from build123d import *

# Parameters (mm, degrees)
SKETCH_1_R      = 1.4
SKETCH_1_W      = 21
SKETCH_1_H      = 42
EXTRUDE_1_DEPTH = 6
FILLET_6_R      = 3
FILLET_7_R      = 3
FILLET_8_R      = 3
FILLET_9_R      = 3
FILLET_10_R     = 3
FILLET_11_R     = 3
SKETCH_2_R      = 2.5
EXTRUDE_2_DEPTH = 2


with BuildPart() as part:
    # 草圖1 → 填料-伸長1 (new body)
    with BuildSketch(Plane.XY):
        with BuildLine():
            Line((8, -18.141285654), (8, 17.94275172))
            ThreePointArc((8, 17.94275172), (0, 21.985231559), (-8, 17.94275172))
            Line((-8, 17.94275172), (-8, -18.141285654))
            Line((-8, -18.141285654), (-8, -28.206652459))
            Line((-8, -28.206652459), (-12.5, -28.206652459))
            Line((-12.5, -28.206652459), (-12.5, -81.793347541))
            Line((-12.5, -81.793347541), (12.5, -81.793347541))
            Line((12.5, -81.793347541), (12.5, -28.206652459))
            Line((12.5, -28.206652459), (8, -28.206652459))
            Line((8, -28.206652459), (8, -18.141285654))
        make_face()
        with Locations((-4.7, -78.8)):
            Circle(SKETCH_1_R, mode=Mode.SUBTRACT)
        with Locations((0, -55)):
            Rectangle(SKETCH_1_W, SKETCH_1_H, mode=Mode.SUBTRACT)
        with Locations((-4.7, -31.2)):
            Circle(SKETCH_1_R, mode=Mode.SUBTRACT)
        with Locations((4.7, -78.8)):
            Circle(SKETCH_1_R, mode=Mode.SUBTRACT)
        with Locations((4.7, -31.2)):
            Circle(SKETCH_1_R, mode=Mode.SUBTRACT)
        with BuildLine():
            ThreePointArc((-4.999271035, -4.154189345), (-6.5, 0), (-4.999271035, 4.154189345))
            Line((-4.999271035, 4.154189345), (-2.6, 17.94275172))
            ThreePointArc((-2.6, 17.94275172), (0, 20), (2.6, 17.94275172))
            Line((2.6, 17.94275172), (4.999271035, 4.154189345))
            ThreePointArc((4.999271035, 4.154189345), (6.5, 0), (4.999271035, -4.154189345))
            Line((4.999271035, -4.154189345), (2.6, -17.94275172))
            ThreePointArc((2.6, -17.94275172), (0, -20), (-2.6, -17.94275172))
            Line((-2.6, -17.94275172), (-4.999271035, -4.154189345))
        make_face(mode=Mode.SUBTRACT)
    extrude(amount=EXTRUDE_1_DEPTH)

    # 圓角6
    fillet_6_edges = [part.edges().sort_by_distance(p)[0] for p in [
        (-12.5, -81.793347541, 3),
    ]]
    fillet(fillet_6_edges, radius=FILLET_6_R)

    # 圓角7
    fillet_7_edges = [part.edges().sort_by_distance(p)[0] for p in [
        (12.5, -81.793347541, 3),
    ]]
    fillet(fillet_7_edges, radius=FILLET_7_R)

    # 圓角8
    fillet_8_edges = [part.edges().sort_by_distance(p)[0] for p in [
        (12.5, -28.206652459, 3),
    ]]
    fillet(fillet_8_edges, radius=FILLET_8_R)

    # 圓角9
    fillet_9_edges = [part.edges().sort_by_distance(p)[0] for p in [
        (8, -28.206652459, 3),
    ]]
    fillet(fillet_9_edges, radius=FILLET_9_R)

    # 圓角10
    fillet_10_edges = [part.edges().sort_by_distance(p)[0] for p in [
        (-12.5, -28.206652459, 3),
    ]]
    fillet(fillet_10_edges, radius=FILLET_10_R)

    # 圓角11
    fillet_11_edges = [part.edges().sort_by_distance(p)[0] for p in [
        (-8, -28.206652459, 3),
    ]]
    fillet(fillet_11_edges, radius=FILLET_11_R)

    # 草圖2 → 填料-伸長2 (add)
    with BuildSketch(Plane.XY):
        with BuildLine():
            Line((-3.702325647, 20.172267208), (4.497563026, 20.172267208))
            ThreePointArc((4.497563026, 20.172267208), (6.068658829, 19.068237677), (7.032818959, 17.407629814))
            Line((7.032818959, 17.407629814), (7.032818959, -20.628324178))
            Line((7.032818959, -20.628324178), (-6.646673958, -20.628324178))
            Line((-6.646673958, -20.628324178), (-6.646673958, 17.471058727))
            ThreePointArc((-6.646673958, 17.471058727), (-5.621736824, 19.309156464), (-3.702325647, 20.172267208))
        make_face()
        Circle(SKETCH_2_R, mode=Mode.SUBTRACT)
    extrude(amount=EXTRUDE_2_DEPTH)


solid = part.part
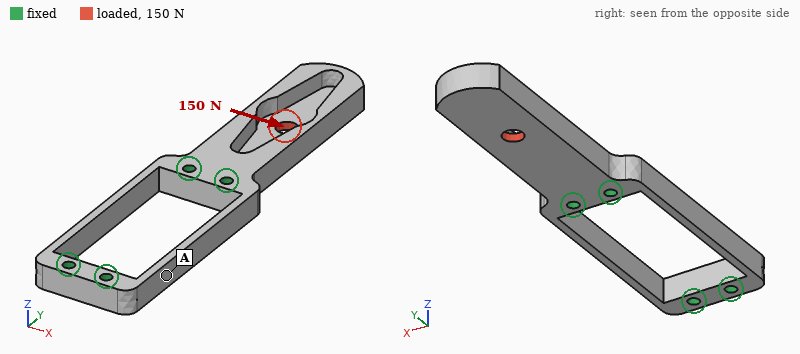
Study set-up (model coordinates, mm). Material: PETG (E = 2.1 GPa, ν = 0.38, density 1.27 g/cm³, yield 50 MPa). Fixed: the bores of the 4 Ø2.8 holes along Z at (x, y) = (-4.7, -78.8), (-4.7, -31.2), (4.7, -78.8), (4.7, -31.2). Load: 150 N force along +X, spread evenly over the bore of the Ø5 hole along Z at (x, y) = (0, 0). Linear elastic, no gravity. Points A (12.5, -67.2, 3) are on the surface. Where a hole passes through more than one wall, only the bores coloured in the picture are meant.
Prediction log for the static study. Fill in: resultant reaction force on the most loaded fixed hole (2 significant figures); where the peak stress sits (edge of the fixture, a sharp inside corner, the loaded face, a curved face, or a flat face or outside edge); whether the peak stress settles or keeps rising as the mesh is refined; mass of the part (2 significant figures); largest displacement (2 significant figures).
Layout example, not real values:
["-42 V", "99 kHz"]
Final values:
["390 N", "edge of the fixture", "keeps rising", "7.5 g", "1.1 mm"]
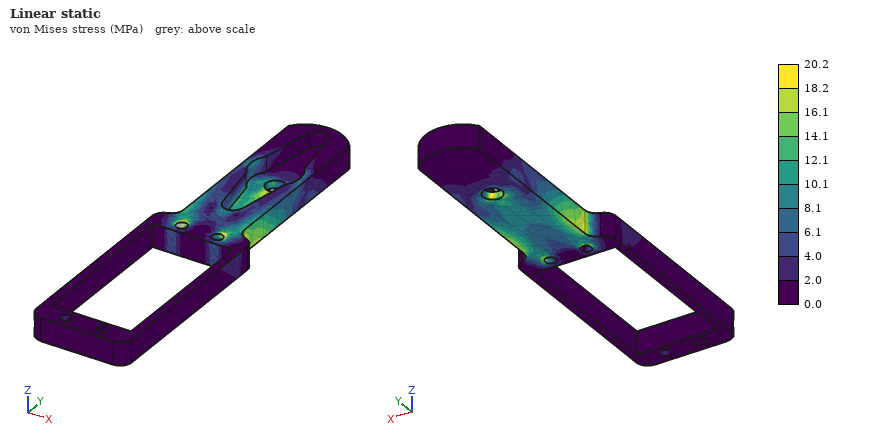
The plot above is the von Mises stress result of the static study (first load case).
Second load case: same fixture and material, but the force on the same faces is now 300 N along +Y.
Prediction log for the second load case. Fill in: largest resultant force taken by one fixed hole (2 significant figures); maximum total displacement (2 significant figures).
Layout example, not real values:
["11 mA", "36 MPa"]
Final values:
["150 N", "1.2 mm"]
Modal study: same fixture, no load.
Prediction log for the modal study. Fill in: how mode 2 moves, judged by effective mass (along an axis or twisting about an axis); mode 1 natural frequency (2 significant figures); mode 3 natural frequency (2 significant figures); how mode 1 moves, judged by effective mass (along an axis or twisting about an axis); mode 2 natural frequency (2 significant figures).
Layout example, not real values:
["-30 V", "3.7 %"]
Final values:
["along X", "500 Hz", "1300 Hz", "along Z", "1100 Hz"]
